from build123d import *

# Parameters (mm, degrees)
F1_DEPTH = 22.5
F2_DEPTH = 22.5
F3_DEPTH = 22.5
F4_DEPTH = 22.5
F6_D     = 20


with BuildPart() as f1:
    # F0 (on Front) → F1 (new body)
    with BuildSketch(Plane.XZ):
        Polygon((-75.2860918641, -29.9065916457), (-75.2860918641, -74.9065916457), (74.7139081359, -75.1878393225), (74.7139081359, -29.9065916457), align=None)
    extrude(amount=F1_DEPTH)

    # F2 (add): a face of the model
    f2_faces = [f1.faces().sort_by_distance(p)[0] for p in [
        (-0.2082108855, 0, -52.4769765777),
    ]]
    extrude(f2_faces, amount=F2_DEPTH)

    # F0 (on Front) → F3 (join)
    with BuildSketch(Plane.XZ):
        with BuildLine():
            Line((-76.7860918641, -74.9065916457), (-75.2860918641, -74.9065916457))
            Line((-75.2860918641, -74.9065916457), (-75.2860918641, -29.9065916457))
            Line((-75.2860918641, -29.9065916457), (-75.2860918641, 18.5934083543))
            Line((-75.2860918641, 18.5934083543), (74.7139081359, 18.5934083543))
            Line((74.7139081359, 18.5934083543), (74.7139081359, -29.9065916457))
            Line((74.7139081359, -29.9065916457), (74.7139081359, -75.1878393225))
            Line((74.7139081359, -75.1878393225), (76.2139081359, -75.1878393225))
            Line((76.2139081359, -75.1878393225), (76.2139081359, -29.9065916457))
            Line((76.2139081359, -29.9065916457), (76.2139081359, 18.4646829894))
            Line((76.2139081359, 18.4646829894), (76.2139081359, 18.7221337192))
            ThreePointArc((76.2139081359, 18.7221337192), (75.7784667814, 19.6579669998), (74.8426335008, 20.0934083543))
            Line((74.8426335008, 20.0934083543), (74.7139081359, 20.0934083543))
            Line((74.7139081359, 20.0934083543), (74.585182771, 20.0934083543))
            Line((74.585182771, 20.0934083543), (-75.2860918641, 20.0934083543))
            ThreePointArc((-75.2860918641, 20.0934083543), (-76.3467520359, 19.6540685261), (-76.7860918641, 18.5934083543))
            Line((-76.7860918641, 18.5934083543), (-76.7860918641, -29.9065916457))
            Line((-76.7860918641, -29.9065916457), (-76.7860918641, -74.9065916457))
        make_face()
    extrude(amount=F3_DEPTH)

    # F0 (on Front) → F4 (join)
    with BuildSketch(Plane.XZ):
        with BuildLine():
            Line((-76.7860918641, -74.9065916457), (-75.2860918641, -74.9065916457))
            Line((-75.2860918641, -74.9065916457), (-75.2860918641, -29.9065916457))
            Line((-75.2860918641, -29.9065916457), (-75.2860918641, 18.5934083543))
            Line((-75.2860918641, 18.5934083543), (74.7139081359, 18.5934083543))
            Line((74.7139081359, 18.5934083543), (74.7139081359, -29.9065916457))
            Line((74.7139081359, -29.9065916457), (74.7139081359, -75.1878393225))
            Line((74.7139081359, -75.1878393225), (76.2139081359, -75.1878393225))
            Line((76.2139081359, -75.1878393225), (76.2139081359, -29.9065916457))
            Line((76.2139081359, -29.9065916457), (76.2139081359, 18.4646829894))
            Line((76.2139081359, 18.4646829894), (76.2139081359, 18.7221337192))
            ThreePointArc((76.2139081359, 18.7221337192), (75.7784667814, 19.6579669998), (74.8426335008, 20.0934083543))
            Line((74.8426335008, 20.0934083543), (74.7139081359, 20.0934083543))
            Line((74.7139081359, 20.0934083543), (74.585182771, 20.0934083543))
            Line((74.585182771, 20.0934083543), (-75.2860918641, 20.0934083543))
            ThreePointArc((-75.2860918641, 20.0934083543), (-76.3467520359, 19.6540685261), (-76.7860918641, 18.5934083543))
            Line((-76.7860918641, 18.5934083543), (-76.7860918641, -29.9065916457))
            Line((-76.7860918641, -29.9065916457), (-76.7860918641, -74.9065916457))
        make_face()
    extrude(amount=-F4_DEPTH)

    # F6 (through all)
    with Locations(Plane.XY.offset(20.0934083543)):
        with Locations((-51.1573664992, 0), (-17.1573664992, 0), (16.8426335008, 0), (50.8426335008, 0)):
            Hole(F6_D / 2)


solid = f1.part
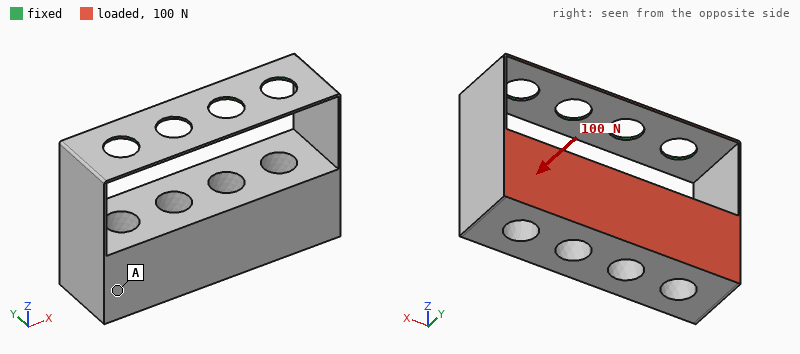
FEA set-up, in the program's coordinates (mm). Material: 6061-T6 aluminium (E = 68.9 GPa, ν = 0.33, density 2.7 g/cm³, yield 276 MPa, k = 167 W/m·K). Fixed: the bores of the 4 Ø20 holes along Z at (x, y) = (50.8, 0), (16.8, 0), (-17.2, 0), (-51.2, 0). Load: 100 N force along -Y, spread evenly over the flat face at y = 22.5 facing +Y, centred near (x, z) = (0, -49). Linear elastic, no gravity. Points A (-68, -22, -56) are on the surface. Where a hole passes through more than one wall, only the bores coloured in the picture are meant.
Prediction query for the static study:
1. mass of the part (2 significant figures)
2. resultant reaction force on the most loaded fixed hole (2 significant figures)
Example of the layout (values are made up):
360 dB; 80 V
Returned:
730 g; 59 N
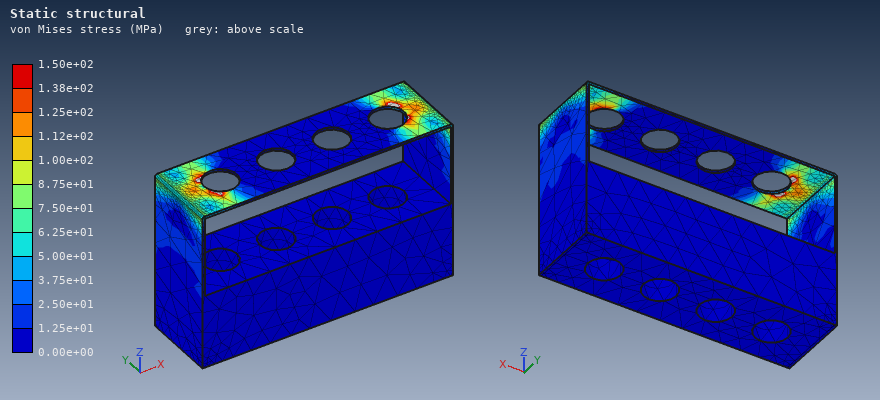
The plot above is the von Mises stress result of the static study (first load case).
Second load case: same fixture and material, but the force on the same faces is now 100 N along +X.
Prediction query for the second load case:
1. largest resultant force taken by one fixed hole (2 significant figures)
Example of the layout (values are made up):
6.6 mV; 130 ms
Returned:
59 N
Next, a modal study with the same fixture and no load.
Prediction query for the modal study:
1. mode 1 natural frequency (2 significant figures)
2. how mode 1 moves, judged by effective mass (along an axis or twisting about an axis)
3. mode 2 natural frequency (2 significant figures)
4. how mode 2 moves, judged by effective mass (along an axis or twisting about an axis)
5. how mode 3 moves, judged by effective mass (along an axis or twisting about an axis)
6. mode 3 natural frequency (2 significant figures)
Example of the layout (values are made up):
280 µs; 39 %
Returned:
46 Hz; along Y; 58 Hz; along X; along Z; 260 Hz
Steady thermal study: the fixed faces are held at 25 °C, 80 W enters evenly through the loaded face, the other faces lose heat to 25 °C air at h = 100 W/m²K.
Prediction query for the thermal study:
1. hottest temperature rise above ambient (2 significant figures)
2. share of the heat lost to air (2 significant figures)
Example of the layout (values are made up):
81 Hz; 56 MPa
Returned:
22 K; 93 %
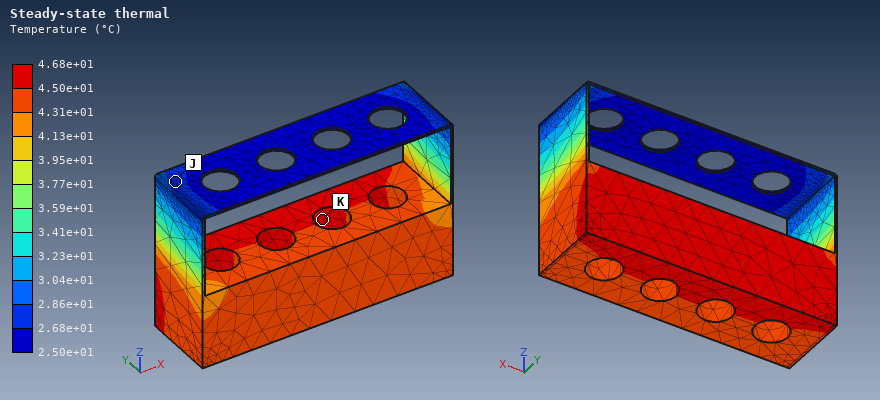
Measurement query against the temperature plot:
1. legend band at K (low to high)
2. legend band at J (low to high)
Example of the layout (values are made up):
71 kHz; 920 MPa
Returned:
4.50e+01 to 4.68e+01 °C; 2.68e+01 to 2.86e+01 °C
